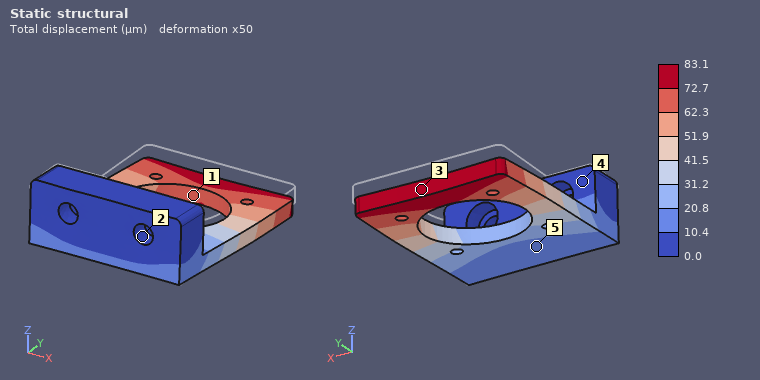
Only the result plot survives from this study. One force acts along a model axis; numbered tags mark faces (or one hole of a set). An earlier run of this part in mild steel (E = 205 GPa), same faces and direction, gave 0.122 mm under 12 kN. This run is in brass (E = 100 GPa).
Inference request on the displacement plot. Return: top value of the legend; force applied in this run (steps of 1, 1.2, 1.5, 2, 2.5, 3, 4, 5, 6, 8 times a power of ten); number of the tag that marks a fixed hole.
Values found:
83.1 µm
4 kN
2
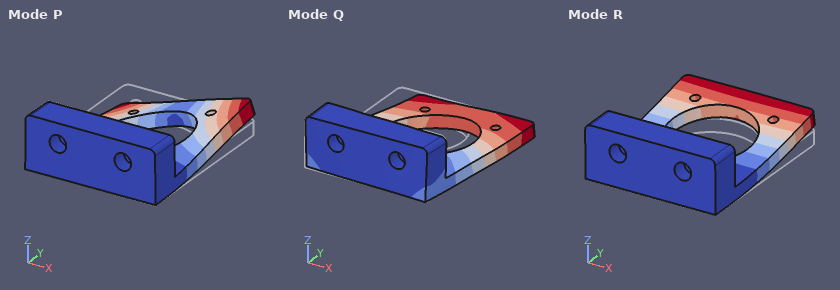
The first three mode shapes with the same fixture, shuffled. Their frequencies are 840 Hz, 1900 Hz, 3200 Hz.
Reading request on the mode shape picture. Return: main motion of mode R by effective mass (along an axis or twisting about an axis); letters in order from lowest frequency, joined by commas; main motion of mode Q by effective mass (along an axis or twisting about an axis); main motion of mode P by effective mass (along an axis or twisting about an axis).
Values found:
along Z
R, P, Q
along X
twisting about Y
